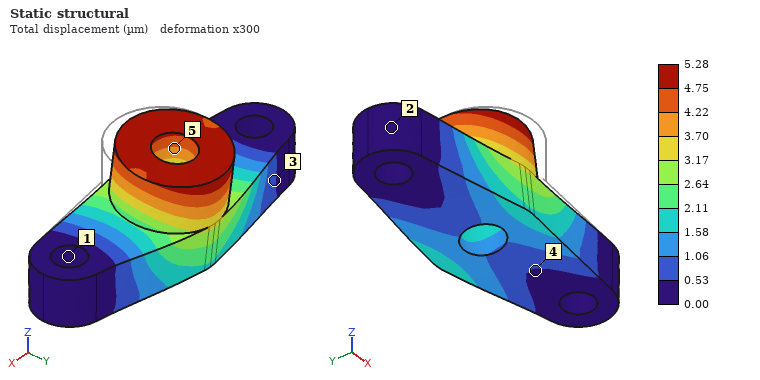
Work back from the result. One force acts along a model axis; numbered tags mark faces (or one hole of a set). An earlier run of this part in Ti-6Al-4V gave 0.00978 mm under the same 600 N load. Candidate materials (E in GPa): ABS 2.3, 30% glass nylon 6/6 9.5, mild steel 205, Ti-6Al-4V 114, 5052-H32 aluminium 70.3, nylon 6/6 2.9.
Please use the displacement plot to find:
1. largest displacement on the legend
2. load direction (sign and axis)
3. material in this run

5.28 µm
+Y
mild steel
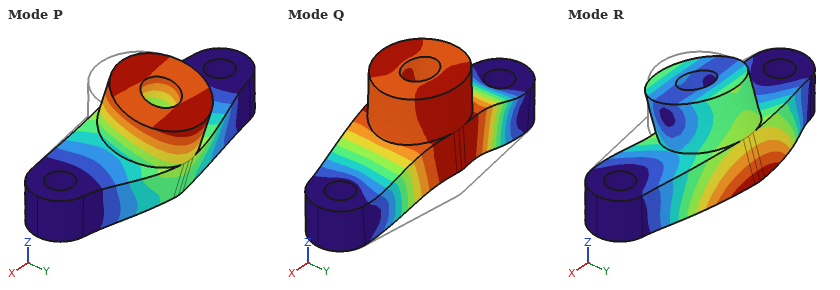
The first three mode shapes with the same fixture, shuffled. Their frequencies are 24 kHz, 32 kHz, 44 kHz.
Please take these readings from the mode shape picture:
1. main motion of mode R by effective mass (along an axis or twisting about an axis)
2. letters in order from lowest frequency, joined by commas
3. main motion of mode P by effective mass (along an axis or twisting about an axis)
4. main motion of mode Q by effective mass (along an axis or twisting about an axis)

along Y
P, Q, R
along Y
along Z
